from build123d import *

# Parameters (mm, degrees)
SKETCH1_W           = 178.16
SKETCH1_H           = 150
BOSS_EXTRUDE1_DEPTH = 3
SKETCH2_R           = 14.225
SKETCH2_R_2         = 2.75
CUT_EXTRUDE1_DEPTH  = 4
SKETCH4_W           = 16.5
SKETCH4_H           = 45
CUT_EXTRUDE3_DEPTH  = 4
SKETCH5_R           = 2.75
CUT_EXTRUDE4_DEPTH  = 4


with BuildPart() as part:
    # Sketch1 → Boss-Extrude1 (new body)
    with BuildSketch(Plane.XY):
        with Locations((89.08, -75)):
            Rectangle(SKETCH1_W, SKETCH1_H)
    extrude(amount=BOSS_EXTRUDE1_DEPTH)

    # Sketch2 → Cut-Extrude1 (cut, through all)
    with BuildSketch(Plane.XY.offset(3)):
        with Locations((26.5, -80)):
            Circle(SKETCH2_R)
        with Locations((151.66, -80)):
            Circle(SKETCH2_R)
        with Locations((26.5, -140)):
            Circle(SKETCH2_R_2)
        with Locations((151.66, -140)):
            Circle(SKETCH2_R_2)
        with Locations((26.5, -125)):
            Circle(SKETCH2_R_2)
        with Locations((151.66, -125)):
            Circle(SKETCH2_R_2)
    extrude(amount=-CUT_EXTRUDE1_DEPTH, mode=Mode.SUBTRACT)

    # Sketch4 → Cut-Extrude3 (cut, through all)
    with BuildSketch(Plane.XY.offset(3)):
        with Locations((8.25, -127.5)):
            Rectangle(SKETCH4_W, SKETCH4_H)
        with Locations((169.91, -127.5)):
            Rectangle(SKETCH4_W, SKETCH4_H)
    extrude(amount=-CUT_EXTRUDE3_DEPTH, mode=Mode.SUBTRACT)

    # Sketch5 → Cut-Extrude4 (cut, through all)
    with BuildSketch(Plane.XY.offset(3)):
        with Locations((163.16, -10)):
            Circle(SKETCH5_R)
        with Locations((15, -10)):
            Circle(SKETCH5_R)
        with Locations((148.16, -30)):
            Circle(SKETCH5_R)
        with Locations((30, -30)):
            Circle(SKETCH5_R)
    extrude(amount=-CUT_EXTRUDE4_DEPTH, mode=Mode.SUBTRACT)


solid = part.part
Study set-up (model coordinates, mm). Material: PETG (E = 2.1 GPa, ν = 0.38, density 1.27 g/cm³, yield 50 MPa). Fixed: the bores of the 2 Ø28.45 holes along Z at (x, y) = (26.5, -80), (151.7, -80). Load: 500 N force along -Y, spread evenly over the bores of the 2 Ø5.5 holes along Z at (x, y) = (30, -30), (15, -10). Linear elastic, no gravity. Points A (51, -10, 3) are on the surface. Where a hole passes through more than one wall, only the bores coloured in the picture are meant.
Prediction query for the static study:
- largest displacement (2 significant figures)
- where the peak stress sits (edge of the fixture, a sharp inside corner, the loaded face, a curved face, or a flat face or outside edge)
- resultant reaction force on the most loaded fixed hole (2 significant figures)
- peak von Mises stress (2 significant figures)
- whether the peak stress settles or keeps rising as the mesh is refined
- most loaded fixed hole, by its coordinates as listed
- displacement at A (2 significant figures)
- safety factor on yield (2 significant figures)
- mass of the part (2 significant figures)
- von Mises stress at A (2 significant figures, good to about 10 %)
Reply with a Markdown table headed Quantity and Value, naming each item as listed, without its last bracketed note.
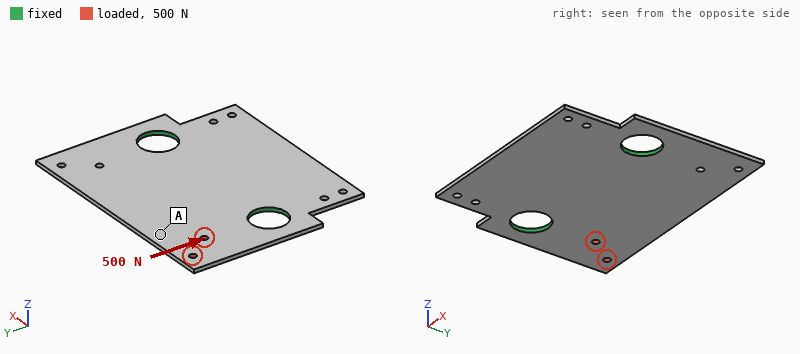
| Quantity | Value |
|---|---|
| largest displacement | 0.13 mm |
| where the peak stress sits | the loaded face |
| resultant reaction force on the most loaded fixed hole | 500 N |
| peak von Mises stress | 11 MPa |
| whether the peak stress settles or keeps rising as the mesh is refined | settles |
| most loaded fixed hole, by its coordinates as listed | (26.5, -80) |
| displacement at A | 0.046 mm |
| safety factor on yield | 4.7 |
| mass of the part | 91 g |
| von Mises stress at A | 0.71 MPa |
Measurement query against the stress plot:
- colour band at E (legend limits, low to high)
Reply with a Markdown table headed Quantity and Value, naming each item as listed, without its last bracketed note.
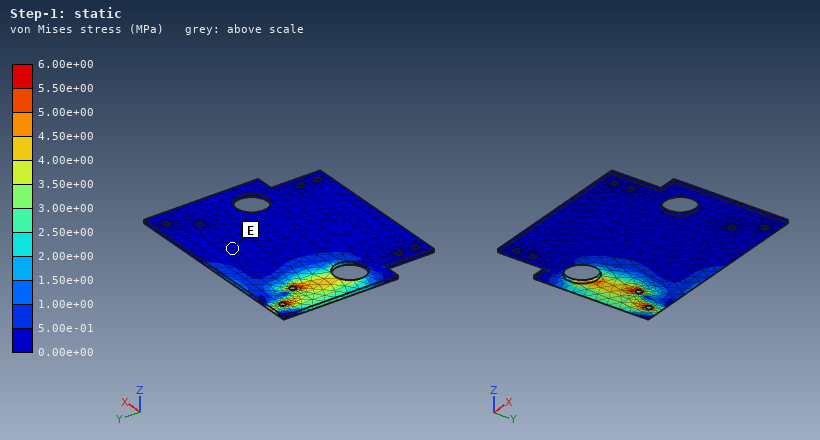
| Quantity | Value |
|---|---|
| colour band at E | 0.00e+00 to 5.00e-01 MPa |
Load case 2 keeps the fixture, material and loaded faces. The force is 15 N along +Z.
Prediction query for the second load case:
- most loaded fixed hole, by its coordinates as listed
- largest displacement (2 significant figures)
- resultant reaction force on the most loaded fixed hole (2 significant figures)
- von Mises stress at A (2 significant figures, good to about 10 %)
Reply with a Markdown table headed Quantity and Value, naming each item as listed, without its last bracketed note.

| Quantity | Value |
|---|---|
| most loaded fixed hole, by its coordinates as listed | (26.5, -80) |
| largest displacement | 2.6 mm |
| resultant reaction force on the most loaded fixed hole | 15 N |
| von Mises stress at A | 1.7 MPa |
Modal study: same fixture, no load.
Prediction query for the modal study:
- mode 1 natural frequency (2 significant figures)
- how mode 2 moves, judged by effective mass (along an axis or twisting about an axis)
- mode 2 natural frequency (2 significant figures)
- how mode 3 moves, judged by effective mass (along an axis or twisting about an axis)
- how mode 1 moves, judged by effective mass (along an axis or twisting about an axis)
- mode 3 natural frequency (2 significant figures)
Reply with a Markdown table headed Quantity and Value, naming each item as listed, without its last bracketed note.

| Quantity | Value |
|---|---|
| mode 1 natural frequency | 120 Hz |
| how mode 2 moves, judged by effective mass | along Z |
| mode 2 natural frequency | 150 Hz |
| how mode 3 moves, judged by effective mass | twisting about Y |
| how mode 1 moves, judged by effective mass | along Z |
| mode 3 natural frequency | 180 Hz |
